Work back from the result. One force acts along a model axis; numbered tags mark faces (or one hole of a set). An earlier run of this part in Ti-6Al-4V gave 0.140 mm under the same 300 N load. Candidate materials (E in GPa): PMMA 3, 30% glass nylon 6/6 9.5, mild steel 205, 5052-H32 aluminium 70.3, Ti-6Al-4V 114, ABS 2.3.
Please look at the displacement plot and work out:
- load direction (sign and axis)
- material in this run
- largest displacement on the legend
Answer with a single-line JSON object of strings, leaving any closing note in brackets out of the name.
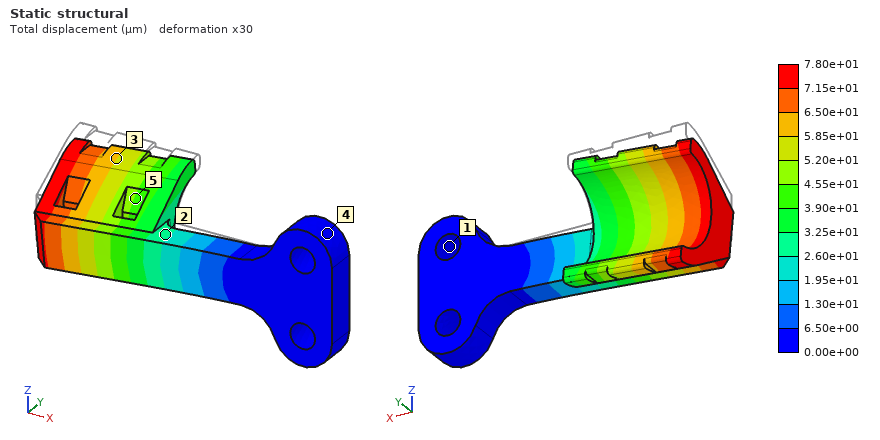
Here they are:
{"load direction": "-Z", "material in this run": "mild steel", "largest displacement on the legend": "7.80e+01 µm"}
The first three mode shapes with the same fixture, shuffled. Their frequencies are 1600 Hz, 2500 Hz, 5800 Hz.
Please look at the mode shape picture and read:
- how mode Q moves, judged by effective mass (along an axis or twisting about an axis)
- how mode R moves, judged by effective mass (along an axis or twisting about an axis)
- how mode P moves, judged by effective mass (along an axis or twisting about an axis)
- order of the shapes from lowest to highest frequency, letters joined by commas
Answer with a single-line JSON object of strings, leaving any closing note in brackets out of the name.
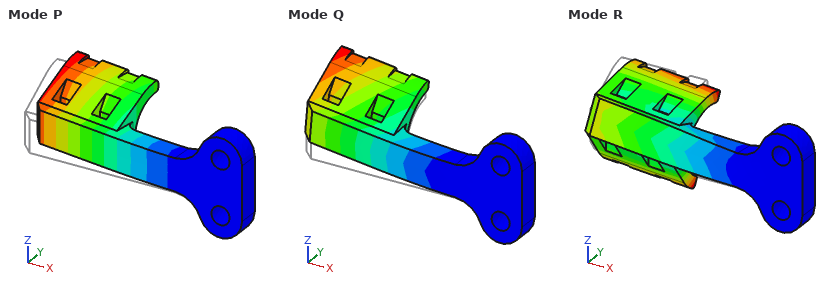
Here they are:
{"how mode Q moves, judged by effective mass": "along Z", "how mode R moves, judged by effective mass": "twisting about X", "how mode P moves, judged by effective mass": "along Y", "order of the shapes from lowest to highest frequency, letters joined by commas": "P, Q, R"}
